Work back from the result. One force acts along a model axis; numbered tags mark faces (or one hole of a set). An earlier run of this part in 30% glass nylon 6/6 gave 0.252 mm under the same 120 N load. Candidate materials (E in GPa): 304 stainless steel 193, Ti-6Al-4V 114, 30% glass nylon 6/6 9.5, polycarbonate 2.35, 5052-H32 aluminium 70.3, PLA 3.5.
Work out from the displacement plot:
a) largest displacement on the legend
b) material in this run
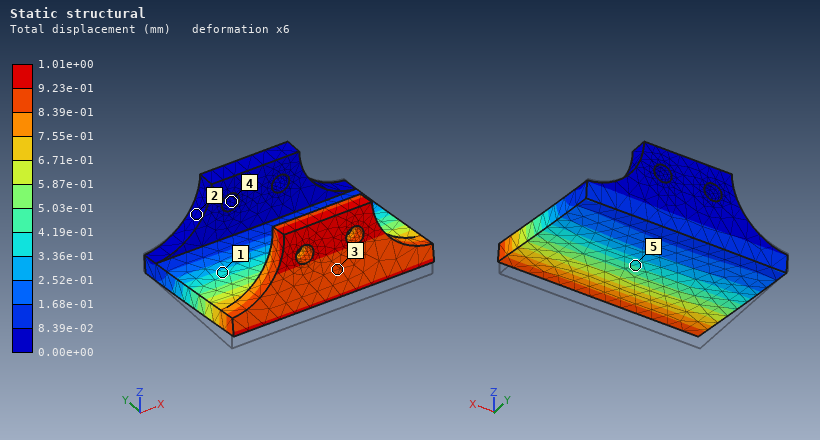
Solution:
1.01e+00 mm
polycarbonate
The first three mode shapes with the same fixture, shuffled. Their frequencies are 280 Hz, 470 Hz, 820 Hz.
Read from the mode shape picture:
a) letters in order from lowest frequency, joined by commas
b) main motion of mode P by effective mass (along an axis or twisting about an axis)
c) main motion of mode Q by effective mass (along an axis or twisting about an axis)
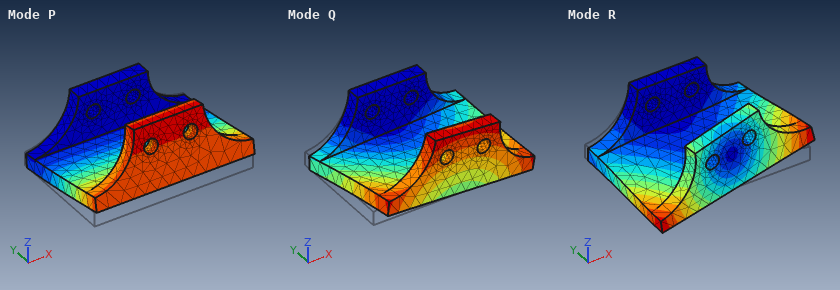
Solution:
P, Q, R
along Z
along X
